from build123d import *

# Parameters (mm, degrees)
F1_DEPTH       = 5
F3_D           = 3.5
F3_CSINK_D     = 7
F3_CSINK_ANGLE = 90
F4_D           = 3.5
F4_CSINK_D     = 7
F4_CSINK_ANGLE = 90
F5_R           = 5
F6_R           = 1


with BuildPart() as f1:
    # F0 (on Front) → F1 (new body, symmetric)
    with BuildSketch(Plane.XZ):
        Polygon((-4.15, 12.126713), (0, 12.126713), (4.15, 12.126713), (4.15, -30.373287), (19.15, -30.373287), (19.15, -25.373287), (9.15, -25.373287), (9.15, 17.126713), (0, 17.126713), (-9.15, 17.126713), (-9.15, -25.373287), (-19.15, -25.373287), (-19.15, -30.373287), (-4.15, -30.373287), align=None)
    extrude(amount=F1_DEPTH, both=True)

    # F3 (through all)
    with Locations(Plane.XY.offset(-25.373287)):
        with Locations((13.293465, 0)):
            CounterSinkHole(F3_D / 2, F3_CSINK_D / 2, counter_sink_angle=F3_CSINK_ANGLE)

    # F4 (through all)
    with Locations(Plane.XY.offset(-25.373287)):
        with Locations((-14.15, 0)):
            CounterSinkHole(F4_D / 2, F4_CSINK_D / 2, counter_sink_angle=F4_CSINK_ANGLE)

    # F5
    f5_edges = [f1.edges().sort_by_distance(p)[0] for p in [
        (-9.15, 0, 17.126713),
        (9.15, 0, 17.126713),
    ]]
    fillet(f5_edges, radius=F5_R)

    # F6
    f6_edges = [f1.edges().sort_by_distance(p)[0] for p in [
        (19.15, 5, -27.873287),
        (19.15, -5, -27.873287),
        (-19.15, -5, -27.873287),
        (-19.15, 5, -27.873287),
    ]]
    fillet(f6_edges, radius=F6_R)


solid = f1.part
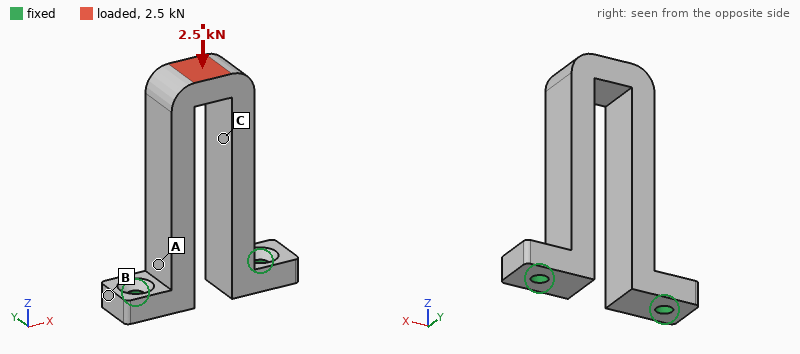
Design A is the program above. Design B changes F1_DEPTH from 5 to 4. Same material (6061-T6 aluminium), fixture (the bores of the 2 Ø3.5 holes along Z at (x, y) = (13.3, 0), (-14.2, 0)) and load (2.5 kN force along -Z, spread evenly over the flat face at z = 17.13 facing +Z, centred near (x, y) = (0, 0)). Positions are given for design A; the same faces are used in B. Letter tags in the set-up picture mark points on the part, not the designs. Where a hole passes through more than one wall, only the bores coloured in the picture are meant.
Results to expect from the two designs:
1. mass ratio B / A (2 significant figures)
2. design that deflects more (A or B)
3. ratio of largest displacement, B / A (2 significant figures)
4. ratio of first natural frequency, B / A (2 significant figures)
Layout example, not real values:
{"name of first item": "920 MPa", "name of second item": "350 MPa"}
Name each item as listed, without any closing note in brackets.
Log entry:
{"mass ratio B / A": "0.80", "design that deflects more": "B", "ratio of largest displacement, B / A": "1.2", "ratio of first natural frequency, B / A": "0.92"}
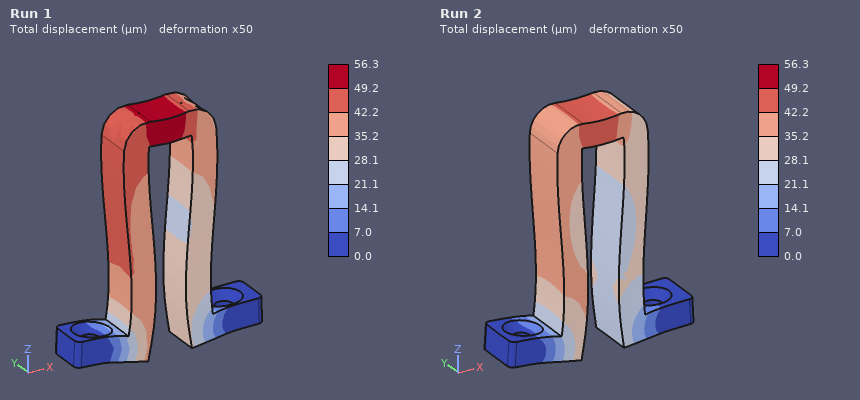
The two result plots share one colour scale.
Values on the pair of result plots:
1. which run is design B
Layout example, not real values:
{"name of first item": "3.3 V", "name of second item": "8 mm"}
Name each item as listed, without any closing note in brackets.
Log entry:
{"which run is design B": "Run 1"}
